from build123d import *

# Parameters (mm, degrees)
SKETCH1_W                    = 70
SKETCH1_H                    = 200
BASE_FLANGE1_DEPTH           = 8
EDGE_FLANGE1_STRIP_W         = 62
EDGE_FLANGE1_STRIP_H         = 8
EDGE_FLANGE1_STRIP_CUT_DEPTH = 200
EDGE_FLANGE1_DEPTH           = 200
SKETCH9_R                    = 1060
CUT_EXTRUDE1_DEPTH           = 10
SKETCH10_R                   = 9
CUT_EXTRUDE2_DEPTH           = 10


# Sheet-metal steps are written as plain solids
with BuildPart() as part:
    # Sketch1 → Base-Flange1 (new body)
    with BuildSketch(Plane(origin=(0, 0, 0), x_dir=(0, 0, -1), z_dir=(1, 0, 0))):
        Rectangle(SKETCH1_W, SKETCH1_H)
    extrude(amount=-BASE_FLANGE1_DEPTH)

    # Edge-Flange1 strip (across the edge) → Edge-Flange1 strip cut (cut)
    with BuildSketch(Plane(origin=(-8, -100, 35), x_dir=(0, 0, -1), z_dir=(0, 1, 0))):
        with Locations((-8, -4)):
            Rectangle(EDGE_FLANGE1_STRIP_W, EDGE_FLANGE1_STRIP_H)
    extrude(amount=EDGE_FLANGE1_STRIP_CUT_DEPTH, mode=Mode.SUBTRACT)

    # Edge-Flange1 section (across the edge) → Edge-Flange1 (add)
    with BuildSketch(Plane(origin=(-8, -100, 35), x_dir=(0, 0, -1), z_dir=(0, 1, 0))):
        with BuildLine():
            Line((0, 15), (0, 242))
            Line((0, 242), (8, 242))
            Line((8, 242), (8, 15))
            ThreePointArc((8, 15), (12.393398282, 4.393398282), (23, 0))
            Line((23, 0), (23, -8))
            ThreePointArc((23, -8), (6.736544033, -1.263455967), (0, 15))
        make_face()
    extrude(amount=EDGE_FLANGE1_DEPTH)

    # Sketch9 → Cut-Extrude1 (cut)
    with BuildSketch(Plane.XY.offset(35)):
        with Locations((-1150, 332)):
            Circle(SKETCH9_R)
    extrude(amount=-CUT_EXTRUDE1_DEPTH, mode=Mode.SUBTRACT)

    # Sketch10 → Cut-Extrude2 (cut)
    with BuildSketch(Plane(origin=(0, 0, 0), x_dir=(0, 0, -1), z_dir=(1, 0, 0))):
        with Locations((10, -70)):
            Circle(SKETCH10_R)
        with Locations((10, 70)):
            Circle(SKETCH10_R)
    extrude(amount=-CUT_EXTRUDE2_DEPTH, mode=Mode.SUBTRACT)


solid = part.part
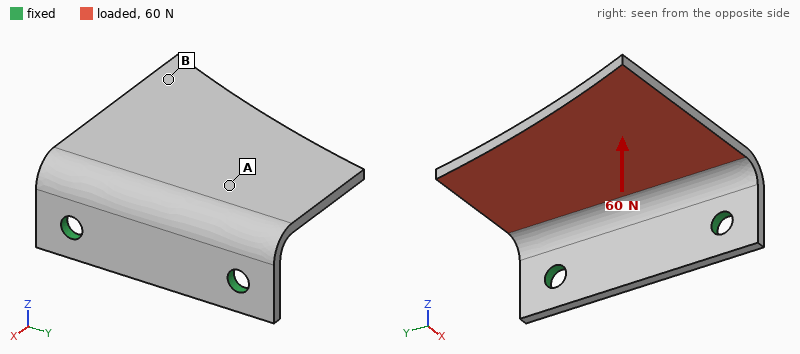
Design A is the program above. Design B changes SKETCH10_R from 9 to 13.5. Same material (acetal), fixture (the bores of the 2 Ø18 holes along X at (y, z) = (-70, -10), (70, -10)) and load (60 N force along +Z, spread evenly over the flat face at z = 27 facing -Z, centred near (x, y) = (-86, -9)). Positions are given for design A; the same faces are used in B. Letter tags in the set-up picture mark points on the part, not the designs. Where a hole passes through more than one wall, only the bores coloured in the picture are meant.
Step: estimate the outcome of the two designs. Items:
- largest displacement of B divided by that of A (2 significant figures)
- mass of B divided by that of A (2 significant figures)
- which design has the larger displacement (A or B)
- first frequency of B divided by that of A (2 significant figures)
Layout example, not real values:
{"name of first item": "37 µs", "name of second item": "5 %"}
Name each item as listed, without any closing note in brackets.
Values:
{"largest displacement of B divided by that of A": "0.91", "mass of B divided by that of A": "0.98", "which design has the larger displacement": "A", "first frequency of B divided by that of A": "1.1"}
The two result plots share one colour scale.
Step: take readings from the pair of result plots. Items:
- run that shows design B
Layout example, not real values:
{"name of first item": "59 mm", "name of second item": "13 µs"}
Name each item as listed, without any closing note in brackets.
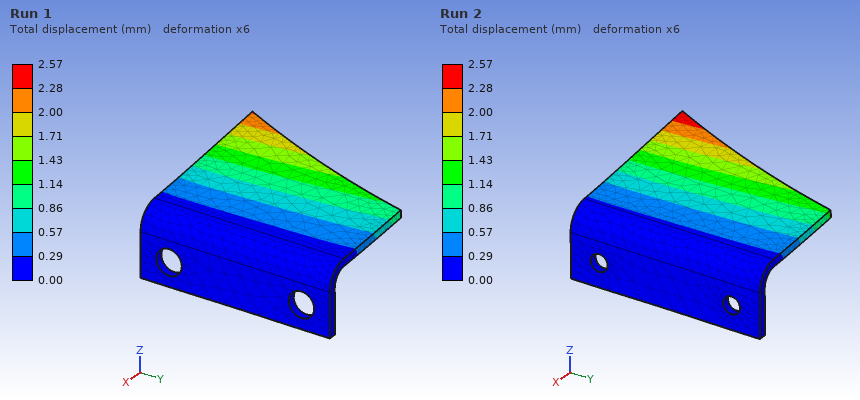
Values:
{"run that shows design B": "Run 1"}
